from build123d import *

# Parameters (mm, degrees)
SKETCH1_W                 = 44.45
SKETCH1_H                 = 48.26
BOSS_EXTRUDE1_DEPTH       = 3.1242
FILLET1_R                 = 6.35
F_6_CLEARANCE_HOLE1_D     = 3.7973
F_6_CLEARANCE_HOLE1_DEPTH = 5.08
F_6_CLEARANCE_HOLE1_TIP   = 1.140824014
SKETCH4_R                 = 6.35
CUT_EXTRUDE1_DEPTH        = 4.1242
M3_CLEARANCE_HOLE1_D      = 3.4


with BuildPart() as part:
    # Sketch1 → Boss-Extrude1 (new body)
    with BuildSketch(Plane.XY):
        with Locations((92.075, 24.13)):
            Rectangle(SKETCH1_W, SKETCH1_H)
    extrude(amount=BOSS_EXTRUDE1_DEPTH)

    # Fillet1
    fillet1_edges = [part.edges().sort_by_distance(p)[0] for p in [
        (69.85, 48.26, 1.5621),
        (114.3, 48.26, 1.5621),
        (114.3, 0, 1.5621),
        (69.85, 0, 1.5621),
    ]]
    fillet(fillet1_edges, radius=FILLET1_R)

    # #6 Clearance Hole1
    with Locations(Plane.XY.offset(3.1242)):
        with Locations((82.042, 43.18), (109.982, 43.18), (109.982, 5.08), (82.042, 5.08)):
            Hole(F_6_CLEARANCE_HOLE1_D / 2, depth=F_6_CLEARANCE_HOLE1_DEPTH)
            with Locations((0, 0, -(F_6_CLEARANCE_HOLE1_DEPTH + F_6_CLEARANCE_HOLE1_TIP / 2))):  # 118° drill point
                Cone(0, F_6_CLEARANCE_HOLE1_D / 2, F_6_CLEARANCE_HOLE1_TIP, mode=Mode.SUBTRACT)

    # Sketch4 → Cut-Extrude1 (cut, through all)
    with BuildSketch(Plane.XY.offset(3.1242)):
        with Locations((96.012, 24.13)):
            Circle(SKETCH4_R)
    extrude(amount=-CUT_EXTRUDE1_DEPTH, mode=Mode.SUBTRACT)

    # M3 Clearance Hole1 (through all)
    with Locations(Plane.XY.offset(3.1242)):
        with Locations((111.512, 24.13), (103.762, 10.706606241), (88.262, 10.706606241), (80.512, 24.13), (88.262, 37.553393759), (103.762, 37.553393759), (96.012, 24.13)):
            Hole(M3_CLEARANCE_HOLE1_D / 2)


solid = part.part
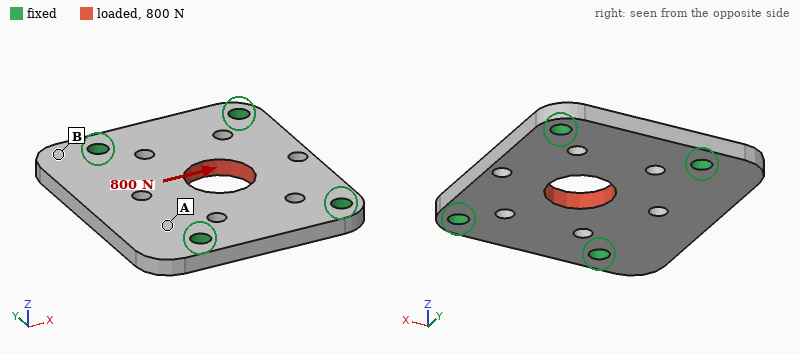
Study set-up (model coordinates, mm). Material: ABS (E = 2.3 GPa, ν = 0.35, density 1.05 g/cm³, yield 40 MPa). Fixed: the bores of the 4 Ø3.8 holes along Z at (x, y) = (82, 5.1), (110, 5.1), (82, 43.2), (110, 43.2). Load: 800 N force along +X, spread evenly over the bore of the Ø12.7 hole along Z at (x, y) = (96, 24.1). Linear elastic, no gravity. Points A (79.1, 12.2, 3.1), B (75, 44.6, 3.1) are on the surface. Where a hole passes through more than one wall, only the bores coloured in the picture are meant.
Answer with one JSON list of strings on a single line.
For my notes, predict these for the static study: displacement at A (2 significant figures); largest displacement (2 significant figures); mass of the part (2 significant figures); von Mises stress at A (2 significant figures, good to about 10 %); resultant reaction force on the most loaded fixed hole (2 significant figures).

["0.035 mm", "0.10 mm", "6.2 g", "4.8 MPa", "240 N"]
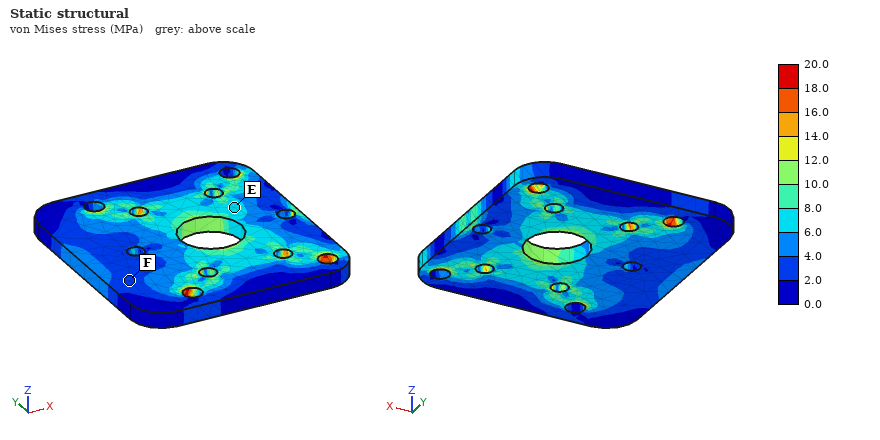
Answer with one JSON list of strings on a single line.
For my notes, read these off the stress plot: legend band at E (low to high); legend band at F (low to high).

["6.0 to 8.0 MPa", "2.0 to 4.0 MPa"]
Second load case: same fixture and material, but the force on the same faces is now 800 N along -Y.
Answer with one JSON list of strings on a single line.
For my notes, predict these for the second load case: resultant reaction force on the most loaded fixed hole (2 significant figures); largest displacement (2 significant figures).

["210 N", "63 µm"]
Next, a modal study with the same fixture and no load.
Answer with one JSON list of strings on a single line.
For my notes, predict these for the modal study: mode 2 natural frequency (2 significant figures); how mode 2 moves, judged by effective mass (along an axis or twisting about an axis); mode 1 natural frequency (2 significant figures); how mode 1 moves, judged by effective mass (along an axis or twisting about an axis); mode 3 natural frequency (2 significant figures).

["3200 Hz", "along Z", "2800 Hz", "along Z", "4500 Hz"]
